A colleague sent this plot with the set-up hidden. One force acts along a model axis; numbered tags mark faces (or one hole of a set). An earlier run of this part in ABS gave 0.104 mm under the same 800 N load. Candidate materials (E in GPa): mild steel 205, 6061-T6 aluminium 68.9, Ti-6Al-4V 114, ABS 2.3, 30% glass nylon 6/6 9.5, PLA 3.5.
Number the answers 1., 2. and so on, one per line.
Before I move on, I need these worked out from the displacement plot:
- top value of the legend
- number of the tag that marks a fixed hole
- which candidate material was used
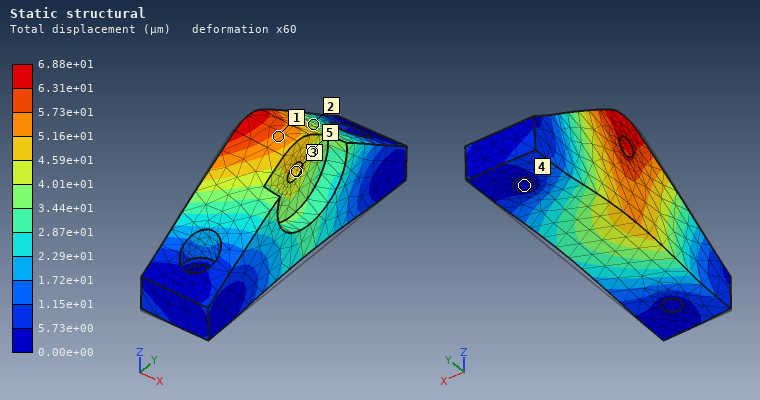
1. 6.88e+01 µm
2. 4
3. PLA
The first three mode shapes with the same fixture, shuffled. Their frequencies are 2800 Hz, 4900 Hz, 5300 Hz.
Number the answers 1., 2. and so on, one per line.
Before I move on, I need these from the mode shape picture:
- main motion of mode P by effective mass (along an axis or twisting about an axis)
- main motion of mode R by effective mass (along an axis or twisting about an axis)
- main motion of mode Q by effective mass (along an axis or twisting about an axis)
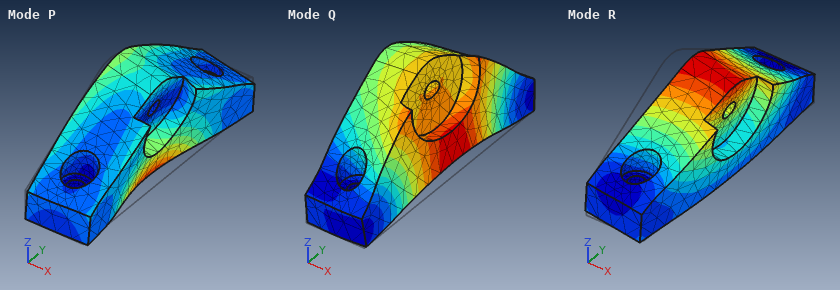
1. along X
2. along X
3. along Z
